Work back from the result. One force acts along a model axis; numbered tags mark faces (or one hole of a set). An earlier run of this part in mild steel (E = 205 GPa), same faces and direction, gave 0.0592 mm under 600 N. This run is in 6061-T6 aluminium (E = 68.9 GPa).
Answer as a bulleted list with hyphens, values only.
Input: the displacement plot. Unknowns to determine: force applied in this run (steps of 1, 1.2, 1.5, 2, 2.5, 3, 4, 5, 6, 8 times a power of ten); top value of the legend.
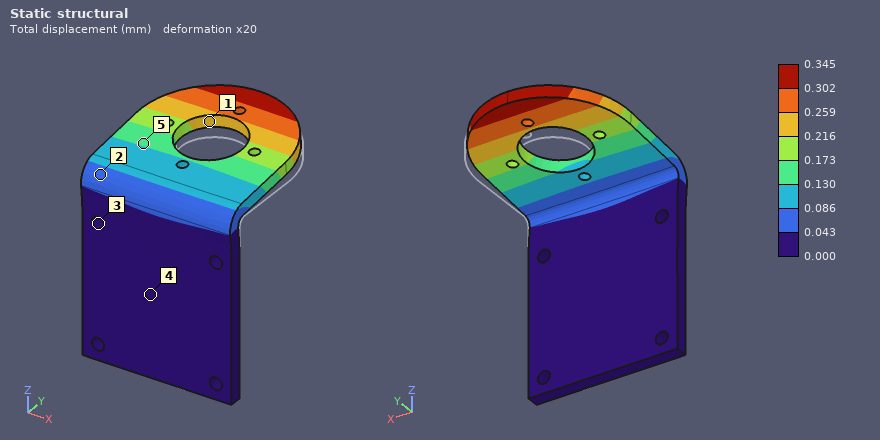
- 1.2 kN
- 0.345 mm
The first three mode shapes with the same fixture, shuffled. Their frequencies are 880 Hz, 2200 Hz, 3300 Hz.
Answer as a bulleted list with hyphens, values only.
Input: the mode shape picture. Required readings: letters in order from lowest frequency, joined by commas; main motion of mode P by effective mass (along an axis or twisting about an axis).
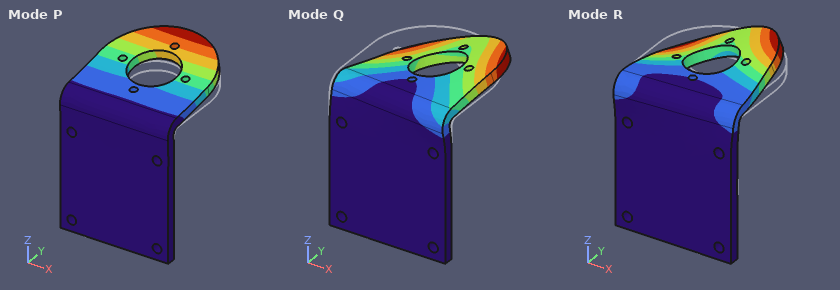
- P, Q, R
- along Z
